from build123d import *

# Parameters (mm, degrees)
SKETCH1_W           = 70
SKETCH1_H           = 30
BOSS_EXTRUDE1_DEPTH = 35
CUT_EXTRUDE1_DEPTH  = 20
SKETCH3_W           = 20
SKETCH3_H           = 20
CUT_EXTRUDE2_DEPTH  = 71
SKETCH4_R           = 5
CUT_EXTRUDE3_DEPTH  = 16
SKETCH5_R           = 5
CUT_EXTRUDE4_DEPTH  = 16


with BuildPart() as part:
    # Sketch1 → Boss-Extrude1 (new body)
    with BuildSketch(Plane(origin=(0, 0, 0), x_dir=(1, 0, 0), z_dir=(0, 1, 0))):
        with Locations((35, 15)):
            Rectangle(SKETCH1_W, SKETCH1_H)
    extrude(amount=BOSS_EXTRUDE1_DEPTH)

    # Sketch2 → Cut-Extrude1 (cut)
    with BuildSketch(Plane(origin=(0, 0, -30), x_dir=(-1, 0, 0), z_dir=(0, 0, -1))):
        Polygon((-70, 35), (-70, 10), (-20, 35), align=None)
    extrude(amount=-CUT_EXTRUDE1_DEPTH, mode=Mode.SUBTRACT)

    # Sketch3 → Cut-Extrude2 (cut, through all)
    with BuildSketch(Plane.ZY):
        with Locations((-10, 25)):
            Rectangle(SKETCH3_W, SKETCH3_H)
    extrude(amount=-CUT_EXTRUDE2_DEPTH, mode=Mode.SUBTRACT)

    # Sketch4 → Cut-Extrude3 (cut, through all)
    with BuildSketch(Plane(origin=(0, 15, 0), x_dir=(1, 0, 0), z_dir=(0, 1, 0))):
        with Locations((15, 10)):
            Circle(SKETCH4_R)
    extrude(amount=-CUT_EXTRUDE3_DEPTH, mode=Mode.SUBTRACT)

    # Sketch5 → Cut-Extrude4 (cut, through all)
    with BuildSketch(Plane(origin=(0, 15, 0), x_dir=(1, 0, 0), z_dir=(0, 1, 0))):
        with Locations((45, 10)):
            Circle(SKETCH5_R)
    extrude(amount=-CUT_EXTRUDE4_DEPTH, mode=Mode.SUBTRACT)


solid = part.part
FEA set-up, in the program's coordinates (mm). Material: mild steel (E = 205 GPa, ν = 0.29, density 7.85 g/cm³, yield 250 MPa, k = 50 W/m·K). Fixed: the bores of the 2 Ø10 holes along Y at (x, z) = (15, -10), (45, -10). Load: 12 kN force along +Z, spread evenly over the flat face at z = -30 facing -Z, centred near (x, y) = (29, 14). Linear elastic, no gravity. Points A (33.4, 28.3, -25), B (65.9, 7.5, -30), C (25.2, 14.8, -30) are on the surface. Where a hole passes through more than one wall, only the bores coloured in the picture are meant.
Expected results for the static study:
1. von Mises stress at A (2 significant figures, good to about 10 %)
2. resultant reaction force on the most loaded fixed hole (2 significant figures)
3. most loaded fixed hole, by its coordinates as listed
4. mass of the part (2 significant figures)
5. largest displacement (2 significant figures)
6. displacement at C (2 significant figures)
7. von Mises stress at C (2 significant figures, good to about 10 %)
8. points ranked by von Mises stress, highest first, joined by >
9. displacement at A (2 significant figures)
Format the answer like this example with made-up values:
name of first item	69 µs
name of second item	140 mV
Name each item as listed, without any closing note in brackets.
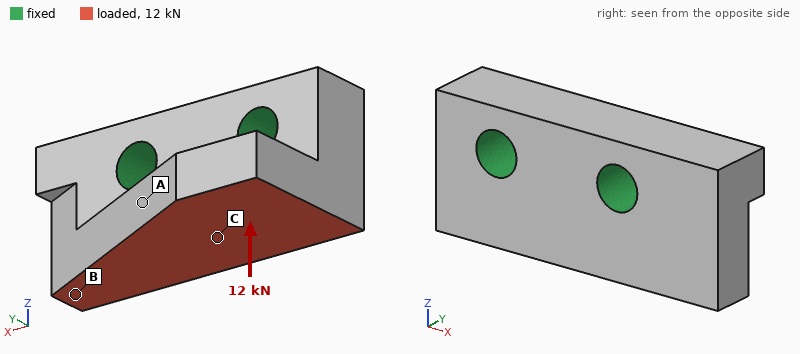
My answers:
von Mises stress at A	25 MPa
resultant reaction force on the most loaded fixed hole	6.6 kN
most loaded fixed hole, by its coordinates as listed	(15, -10)
mass of the part	290 g
largest displacement	28 µm
displacement at C	7.1 µm
von Mises stress at C	49 MPa
points ranked by von Mises stress, highest first, joined by >	C > A > B
displacement at A	13 µm
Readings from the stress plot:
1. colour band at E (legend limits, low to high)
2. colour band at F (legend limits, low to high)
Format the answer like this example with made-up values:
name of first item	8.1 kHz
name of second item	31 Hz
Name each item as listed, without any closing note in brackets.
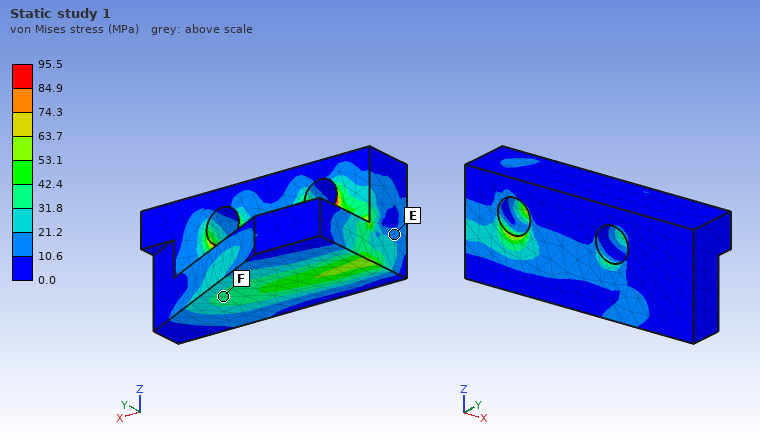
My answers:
colour band at E	10.6 to 21.2 MPa
colour band at F	31.8 to 42.4 MPa
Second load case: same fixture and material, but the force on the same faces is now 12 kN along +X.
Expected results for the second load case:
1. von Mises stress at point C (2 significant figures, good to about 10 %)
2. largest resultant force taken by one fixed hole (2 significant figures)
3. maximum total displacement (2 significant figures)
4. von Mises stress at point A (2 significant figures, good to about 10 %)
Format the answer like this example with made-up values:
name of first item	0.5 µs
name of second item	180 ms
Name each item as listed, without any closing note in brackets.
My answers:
von Mises stress at point C	22 MPa
largest resultant force taken by one fixed hole	8.4 kN
maximum total displacement	11 µm
von Mises stress at point A	18 MPa
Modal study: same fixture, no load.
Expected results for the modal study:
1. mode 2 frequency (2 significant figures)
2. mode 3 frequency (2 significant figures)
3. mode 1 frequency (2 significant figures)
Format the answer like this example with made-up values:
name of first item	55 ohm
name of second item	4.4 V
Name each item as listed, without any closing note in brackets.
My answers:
mode 2 frequency	16 kHz
mode 3 frequency	19 kHz
mode 1 frequency	11 kHz
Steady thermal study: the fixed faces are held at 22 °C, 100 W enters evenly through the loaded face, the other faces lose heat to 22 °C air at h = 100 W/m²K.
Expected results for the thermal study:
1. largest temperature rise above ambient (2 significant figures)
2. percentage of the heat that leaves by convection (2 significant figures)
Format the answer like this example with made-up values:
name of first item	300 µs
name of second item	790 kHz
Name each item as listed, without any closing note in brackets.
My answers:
largest temperature rise above ambient	51 K
percentage of the heat that leaves by convection	11 %
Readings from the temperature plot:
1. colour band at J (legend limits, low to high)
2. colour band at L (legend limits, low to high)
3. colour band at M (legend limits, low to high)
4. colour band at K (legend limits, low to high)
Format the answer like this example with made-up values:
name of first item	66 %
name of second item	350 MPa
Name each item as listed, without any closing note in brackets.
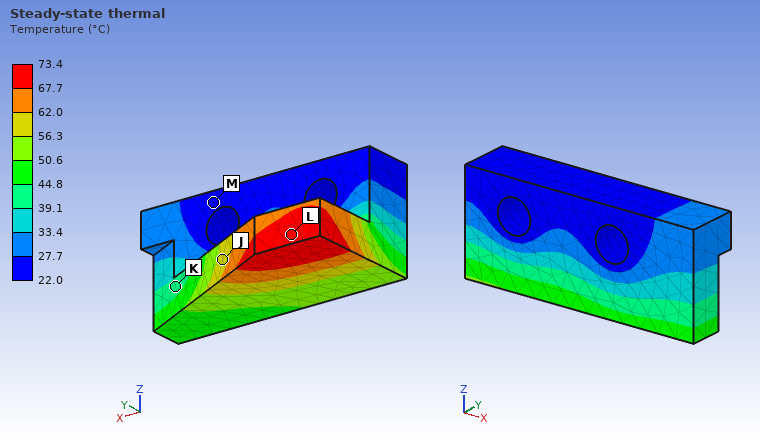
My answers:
colour band at J	56.3 to 62.0 °C
colour band at L	67.7 to 73.4 °C
colour band at M	22.0 to 27.7 °C
colour band at K	39.1 to 44.8 °C
